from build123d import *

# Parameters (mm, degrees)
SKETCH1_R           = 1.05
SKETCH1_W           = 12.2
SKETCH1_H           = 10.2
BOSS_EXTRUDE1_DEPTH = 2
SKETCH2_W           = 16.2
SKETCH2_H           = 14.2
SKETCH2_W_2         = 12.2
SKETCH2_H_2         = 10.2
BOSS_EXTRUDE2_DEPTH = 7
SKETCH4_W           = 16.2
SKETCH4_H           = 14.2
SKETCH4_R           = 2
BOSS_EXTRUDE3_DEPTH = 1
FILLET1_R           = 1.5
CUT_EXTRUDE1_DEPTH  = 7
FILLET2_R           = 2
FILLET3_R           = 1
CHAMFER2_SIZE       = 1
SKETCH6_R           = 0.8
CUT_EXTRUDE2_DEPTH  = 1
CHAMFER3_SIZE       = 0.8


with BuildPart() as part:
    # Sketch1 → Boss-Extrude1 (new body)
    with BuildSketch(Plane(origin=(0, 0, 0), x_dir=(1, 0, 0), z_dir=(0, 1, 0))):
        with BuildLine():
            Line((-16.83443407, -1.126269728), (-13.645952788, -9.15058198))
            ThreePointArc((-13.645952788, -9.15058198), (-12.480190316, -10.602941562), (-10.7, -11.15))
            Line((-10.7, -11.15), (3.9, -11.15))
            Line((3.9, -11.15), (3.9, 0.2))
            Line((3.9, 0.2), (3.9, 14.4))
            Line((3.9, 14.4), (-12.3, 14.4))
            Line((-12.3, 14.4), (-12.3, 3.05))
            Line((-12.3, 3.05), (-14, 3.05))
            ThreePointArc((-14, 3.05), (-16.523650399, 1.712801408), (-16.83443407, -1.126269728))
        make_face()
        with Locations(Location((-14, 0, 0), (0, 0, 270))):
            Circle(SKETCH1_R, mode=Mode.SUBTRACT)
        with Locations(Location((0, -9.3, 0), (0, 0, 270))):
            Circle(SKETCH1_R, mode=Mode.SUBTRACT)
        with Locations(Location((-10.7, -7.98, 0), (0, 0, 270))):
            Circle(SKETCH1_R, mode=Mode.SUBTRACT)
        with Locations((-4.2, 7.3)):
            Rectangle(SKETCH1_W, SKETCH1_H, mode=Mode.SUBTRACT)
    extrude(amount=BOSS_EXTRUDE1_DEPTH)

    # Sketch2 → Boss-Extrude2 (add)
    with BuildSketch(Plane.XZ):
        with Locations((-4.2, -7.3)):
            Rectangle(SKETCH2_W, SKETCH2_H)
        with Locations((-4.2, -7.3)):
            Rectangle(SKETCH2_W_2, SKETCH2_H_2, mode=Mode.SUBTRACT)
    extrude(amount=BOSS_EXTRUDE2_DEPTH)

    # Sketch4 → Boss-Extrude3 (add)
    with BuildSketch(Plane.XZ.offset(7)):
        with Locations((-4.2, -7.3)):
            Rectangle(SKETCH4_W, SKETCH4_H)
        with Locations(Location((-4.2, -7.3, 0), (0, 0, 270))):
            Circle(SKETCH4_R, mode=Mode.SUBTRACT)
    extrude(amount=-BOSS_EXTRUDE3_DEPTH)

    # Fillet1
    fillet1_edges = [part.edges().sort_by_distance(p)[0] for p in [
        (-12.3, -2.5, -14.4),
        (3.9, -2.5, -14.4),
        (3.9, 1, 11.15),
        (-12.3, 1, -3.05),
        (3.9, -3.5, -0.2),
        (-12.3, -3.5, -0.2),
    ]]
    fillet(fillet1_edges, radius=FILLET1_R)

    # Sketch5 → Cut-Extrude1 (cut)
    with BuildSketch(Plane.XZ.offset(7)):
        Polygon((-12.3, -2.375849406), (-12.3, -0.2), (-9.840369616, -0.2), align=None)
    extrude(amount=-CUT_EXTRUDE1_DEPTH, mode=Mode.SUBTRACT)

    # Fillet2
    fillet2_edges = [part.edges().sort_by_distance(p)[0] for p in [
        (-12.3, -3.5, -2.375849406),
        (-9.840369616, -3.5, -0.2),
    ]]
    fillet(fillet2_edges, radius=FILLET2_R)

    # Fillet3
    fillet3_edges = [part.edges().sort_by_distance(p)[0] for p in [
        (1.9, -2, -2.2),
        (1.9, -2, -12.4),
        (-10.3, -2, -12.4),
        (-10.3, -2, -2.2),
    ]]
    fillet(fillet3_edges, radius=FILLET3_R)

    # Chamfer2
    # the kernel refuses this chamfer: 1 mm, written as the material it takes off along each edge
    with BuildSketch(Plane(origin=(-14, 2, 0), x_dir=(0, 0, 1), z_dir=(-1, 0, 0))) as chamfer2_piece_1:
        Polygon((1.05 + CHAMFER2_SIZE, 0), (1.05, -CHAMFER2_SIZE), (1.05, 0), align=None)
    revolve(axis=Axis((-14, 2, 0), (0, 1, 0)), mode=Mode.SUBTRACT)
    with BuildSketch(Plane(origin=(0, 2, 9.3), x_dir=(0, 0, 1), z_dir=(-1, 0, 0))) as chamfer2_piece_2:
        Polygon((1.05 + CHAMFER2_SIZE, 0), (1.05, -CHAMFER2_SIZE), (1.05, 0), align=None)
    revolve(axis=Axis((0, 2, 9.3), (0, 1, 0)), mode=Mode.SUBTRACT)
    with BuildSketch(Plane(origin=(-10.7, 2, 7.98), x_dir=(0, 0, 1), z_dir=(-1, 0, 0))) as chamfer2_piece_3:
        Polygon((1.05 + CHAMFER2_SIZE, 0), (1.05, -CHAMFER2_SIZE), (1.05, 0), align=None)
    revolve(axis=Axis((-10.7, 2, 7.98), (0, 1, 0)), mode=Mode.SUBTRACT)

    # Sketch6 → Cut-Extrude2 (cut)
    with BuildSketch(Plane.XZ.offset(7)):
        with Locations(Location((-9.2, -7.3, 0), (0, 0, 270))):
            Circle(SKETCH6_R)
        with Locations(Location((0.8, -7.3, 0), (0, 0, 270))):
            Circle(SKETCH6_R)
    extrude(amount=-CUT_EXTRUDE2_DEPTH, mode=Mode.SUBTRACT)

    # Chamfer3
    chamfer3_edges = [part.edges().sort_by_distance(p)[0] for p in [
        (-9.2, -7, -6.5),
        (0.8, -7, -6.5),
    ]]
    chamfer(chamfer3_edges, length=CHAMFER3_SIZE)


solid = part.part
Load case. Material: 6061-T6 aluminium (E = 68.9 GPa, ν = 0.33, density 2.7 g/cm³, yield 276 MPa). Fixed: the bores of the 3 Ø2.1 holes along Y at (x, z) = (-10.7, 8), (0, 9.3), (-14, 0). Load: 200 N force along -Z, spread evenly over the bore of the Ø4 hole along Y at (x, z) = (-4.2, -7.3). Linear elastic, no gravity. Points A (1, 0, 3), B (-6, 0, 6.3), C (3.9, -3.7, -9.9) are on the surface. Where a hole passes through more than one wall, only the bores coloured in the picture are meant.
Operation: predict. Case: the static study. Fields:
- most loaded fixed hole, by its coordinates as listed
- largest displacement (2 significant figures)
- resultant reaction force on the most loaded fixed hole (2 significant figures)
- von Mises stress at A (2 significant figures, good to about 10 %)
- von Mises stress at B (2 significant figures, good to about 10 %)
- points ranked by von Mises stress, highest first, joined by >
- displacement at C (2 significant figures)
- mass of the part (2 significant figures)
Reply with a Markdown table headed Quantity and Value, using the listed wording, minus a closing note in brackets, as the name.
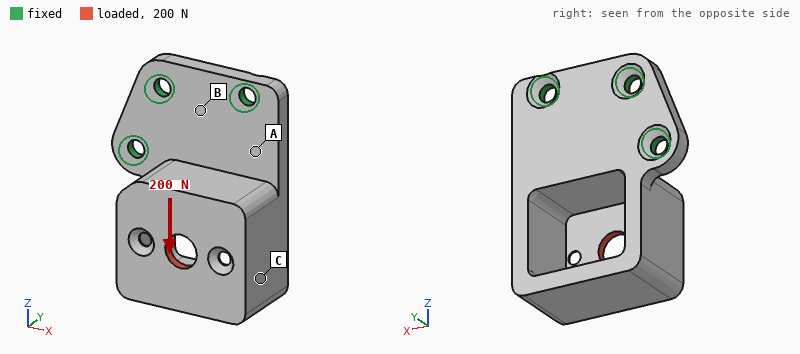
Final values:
| Quantity | Value |
|---|---|
| most loaded fixed hole, by its coordinates as listed | (0, 9.3) |
| largest displacement | 0.22 mm |
| resultant reaction force on the most loaded fixed hole | 140 N |
| von Mises stress at A | 73 MPa |
| von Mises stress at B | 38 MPa |
| points ranked by von Mises stress, highest first, joined by > | A > B > C |
| displacement at C | 0.17 mm |
| mass of the part | 3.9 g |
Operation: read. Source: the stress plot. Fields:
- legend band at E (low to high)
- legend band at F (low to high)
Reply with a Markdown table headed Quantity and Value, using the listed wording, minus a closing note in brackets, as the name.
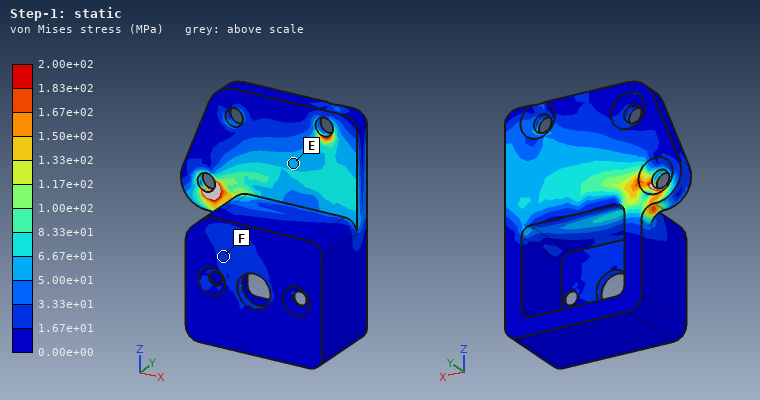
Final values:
| Quantity | Value |
|---|---|
| legend band at E | 5.00e+01 to 6.67e+01 MPa |
| legend band at F | 1.67e+01 to 3.33e+01 MPa |
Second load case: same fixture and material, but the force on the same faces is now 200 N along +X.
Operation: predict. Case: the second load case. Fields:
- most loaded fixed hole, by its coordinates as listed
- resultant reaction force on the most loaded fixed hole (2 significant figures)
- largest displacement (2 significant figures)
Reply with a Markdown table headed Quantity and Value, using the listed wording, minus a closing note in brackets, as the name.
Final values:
| Quantity | Value |
|---|---|
| most loaded fixed hole, by its coordinates as listed | (-14, 0) |
| resultant reaction force on the most loaded fixed hole | 240 N |
| largest displacement | 0.12 mm |
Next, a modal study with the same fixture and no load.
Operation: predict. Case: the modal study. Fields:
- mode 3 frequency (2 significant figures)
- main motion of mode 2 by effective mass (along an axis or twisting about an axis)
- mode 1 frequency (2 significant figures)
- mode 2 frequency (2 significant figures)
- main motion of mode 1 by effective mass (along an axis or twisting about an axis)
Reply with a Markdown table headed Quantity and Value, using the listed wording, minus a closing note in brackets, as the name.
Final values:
| Quantity | Value |
|---|---|
| mode 3 frequency | 9300 Hz |
| main motion of mode 2 by effective mass | along X |
| mode 1 frequency | 2800 Hz |
| mode 2 frequency | 8900 Hz |
| main motion of mode 1 by effective mass | along Y |
